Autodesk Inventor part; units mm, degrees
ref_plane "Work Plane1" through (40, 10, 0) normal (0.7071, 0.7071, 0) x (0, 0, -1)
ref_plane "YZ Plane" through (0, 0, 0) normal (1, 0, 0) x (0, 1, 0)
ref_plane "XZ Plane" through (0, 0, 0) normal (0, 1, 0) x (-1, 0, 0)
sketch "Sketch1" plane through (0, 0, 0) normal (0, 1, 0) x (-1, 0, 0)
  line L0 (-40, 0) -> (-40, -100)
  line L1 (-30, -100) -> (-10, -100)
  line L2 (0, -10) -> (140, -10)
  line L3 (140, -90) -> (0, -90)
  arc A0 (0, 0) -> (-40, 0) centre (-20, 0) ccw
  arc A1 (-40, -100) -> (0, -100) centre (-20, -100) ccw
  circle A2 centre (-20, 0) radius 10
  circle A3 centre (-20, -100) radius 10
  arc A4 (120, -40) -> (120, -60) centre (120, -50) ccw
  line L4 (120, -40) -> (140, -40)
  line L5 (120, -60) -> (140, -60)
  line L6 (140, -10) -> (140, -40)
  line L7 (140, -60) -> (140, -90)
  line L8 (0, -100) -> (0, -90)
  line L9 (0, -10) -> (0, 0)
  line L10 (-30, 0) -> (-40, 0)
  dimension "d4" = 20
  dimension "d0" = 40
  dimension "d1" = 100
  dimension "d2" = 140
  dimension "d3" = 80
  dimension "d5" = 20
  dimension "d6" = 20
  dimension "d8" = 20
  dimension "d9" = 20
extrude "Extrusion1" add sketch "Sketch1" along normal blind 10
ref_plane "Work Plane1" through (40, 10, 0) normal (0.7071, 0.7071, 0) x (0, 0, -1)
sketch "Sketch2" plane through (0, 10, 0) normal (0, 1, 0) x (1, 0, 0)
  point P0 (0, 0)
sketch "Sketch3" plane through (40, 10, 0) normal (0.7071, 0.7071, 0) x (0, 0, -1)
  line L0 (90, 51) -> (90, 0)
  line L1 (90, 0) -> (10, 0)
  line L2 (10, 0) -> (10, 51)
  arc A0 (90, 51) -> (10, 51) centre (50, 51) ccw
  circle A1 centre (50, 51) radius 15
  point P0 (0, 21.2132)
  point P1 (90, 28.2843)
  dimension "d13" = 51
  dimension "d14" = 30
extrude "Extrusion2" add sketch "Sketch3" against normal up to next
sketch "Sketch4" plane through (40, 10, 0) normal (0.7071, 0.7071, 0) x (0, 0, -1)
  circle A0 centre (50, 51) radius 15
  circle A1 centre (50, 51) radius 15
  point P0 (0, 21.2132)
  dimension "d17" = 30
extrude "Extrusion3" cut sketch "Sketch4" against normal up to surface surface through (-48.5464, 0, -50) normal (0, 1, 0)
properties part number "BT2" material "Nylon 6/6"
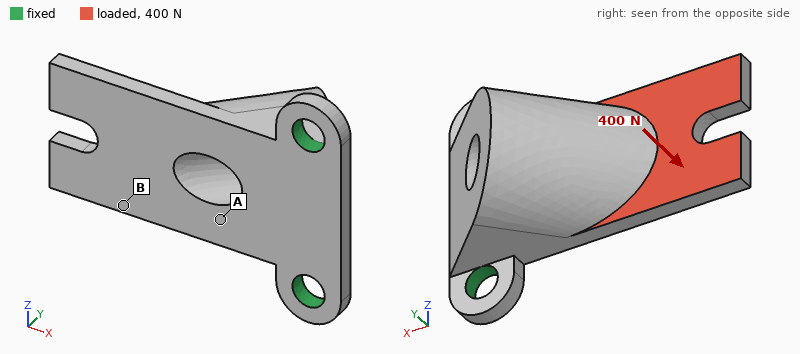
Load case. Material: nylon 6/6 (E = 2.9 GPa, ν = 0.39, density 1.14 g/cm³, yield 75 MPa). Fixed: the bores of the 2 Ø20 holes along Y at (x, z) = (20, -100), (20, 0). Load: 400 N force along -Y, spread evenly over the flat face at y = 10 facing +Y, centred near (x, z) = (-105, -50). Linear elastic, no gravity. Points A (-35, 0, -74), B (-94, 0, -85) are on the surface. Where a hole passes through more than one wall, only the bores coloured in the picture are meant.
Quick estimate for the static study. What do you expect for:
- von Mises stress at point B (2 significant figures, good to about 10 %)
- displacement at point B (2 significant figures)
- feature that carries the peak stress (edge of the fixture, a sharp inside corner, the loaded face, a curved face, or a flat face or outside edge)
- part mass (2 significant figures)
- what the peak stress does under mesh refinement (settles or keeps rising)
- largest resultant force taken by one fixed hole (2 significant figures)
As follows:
3.6 MPa
1.3 mm
edge of the fixture
430 g
keeps rising
300 N
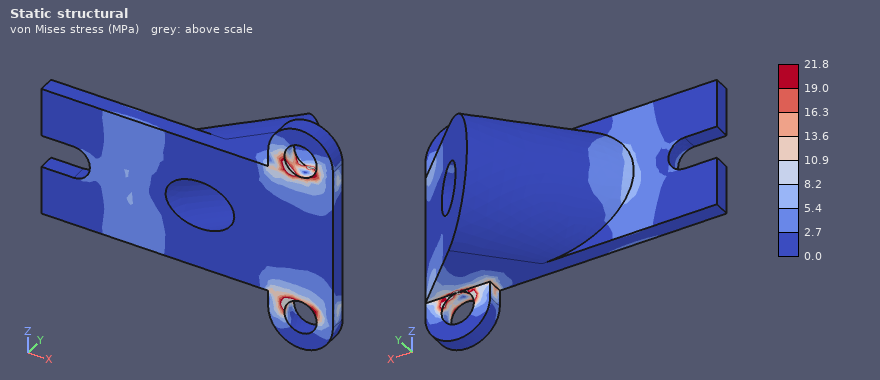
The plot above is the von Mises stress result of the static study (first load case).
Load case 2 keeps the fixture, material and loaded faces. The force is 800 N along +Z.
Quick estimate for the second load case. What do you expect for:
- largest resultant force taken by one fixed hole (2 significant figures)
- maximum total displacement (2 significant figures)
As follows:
1.2 kN
0.46 mm
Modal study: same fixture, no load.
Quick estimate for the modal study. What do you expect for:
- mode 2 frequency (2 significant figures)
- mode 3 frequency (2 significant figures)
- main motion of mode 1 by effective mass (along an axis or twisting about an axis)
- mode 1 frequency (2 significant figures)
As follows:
790 Hz
850 Hz
along Y
250 Hz
